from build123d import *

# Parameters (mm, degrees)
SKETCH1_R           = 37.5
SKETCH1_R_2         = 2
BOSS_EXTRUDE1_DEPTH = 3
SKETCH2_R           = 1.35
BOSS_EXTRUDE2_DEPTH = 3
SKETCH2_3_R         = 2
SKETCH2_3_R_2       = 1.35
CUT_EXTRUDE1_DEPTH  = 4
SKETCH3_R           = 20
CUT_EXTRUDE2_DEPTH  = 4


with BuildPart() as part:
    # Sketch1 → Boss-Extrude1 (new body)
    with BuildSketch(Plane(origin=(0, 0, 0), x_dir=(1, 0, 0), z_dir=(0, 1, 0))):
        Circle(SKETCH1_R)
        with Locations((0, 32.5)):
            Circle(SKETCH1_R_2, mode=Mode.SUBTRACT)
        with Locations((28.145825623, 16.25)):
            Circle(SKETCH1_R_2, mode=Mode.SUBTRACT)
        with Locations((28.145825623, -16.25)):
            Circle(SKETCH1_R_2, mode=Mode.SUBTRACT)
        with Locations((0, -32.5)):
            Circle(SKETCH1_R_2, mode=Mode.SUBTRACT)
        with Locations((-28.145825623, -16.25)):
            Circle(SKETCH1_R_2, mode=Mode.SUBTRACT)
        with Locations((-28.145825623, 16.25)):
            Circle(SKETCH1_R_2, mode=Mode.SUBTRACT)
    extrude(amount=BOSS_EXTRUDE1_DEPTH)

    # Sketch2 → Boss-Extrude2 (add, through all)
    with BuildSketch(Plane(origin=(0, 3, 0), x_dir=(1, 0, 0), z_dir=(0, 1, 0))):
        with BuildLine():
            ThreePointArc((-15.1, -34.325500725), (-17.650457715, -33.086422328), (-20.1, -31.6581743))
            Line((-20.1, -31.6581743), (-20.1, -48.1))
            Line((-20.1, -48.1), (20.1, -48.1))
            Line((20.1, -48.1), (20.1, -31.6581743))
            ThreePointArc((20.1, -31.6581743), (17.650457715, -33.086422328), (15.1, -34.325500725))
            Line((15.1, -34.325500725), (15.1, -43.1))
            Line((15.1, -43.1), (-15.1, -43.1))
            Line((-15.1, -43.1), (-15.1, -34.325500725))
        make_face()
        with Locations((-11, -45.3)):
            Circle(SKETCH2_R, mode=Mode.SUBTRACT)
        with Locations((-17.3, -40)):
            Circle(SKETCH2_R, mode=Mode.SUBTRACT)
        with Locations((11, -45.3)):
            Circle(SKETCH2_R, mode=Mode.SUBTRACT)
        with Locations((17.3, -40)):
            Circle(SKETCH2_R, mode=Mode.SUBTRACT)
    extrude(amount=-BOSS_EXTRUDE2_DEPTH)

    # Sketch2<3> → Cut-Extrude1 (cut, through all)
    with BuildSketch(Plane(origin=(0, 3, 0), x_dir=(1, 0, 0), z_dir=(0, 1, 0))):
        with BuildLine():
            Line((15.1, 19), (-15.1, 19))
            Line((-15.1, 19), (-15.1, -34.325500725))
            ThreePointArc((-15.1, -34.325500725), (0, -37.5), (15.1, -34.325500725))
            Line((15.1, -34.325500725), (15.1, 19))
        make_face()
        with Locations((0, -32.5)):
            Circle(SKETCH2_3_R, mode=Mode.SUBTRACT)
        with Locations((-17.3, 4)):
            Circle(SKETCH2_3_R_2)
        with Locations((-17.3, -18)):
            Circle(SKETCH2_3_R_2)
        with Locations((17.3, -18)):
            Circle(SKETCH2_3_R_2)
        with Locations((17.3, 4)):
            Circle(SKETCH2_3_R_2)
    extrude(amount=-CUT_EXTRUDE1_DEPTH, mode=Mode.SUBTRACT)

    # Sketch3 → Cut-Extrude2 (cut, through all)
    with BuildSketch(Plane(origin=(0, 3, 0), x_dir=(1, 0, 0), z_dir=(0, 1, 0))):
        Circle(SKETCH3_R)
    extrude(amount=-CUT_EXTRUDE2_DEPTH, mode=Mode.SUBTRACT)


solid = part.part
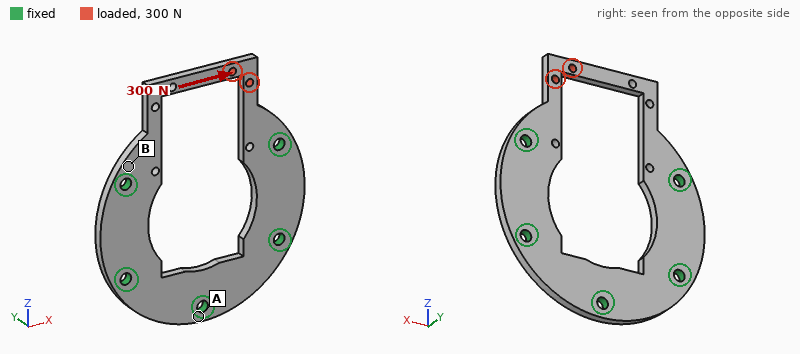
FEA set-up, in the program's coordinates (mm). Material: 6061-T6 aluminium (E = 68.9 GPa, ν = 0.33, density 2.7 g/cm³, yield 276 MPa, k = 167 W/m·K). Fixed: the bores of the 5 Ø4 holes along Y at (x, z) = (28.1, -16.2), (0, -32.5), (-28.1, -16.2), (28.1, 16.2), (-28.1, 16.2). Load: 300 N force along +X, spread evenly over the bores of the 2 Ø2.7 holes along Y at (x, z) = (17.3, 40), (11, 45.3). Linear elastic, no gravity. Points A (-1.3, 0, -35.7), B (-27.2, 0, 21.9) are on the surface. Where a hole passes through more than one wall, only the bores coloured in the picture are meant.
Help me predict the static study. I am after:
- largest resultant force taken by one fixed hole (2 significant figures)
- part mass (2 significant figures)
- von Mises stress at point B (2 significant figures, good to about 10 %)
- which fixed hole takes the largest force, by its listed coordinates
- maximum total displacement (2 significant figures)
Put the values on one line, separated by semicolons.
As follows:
270 N; 22 g; 16 MPa; (28.1, 16.2); 67 µm
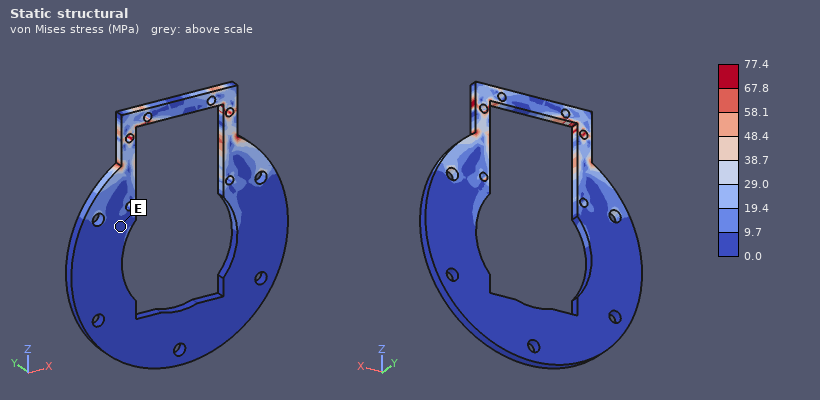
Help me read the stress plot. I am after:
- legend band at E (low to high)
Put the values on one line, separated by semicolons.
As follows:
0.0 to 9.7 MPa
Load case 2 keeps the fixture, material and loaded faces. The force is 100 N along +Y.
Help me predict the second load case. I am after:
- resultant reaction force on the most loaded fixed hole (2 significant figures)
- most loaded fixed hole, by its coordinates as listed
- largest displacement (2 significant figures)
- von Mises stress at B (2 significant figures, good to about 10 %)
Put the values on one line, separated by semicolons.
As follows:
93 N; (28.1, 16.2); 0.41 mm; 32 MPa
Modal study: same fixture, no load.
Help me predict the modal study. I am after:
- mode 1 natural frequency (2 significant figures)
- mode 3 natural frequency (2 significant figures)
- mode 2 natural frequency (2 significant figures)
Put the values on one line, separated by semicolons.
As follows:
2000 Hz; 7500 Hz; 4000 Hz
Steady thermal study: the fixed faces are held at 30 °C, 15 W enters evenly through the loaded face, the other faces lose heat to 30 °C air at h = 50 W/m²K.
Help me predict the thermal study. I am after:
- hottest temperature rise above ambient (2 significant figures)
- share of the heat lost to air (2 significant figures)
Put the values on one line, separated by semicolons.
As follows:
81 K; 20 %
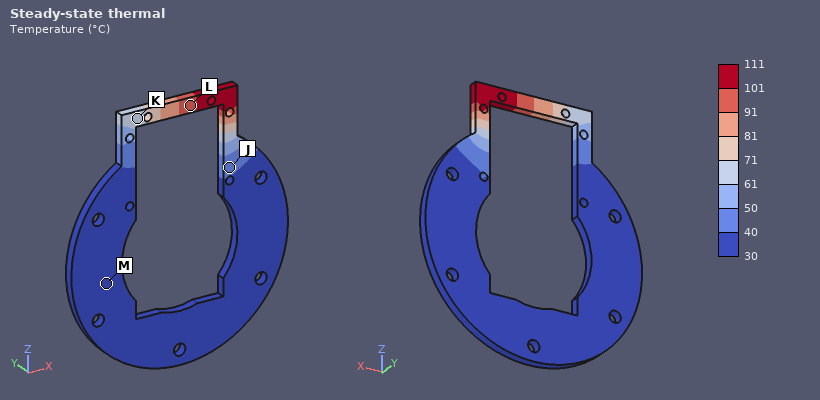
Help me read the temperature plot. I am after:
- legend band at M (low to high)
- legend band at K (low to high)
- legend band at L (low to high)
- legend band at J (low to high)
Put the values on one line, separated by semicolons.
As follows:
30 to 40 °C; 61 to 71 °C; 91 to 101 °C; 40 to 50 °C
